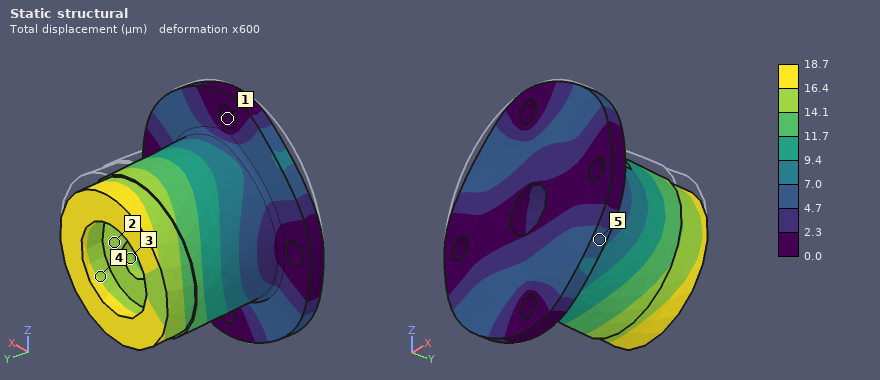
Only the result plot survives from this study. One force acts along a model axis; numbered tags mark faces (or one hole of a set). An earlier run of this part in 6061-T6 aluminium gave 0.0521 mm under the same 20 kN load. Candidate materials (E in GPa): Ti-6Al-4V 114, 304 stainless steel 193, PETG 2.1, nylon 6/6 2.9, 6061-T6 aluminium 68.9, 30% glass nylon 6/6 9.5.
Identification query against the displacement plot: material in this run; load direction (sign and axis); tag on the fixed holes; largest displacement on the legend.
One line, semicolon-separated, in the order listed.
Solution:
304 stainless steel; -Z; 1; 18.7 µm
